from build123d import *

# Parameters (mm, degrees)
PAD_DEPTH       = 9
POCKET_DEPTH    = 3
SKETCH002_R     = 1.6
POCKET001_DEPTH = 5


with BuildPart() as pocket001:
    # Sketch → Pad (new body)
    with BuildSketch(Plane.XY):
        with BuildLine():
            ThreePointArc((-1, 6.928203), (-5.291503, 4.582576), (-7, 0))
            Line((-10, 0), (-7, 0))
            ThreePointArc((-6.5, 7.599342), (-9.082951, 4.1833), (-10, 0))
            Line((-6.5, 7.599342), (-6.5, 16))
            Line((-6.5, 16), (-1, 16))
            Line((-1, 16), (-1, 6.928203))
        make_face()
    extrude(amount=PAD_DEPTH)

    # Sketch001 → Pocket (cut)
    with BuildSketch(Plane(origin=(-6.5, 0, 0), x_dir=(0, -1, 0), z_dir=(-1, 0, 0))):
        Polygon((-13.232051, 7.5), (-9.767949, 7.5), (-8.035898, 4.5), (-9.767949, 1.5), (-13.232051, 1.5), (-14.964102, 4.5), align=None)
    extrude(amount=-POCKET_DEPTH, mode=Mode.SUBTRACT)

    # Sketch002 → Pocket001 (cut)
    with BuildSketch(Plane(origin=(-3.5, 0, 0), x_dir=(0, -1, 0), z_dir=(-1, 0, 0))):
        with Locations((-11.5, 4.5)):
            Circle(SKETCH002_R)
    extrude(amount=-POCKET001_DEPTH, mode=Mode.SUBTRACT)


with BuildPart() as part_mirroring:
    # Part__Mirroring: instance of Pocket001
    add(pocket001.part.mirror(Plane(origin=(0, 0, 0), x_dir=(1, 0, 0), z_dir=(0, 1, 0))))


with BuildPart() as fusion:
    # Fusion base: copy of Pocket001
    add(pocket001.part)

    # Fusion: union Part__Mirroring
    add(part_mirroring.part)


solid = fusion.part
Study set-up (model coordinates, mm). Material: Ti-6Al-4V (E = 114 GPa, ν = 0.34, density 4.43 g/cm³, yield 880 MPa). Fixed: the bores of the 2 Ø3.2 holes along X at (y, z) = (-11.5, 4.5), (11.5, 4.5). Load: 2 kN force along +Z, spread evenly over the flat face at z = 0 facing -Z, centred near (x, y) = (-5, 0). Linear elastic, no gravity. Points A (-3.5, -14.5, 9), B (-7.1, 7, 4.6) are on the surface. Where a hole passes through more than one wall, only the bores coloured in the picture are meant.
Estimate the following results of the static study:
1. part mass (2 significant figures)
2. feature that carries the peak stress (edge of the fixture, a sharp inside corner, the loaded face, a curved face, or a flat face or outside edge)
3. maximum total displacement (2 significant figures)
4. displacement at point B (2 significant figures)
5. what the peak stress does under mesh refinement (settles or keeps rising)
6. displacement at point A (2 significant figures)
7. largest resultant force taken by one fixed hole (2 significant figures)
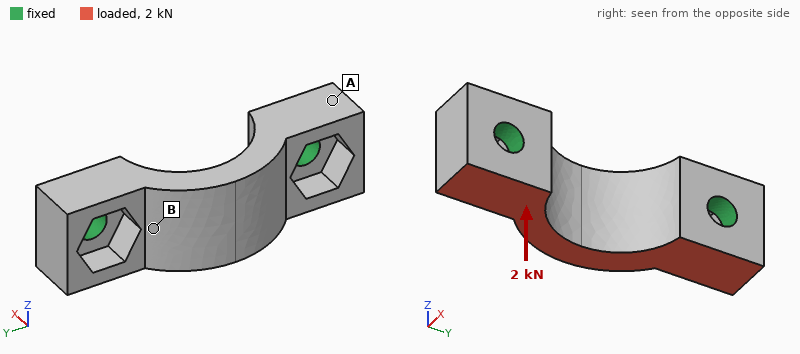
5.0 g
edge of the fixture
25 µm
13 µm
keeps rising
4.3 µm
1.0 kN
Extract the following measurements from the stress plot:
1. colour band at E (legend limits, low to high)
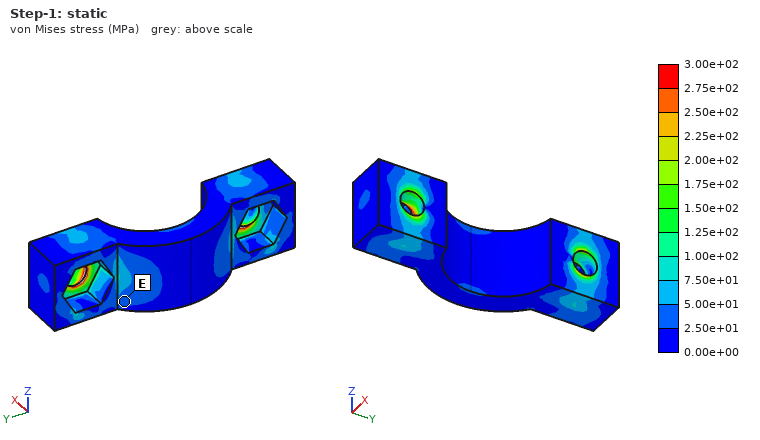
2.50e+01 to 5.00e+01 MPa
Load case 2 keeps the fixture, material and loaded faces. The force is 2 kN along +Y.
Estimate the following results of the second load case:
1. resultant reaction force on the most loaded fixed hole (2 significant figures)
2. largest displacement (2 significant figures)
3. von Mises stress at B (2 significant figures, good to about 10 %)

1.0 kN
11 µm
30 MPa
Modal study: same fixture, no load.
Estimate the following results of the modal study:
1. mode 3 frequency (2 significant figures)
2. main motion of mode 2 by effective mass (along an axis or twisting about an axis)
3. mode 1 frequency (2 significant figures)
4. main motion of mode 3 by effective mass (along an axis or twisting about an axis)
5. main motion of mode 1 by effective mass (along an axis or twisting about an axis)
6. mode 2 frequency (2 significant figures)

48 kHz
along Y
23 kHz
along X
along Z
44 kHz
